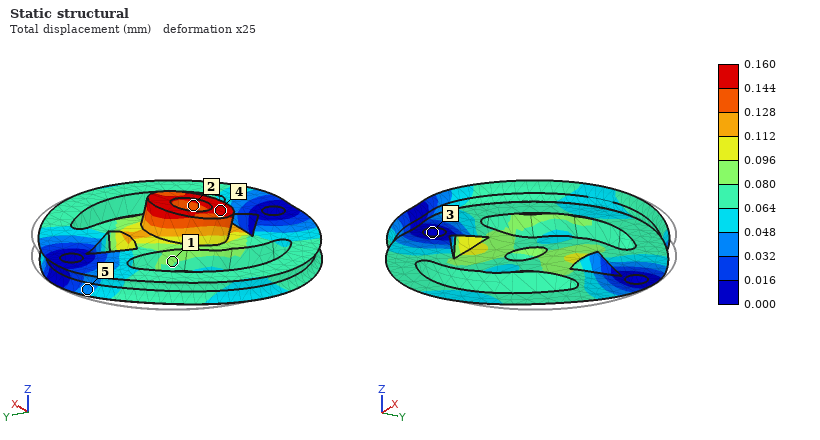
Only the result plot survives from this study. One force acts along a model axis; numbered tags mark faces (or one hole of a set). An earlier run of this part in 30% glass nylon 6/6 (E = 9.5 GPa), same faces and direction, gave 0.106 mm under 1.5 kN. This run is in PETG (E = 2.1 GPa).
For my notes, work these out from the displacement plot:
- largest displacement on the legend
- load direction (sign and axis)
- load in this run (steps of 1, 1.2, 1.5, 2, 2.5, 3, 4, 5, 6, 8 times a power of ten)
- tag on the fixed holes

0.160 mm
-Y
500 N
3
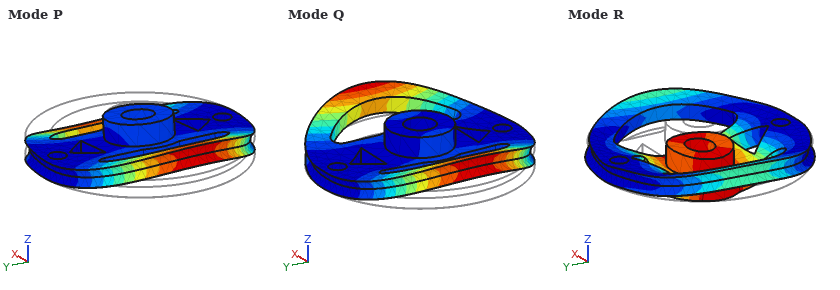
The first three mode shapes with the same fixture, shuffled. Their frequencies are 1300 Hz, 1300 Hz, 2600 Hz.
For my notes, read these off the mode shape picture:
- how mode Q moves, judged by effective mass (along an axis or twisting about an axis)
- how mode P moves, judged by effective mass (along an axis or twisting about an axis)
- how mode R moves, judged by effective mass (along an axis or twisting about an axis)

along Z
twisting about Y
along Z
